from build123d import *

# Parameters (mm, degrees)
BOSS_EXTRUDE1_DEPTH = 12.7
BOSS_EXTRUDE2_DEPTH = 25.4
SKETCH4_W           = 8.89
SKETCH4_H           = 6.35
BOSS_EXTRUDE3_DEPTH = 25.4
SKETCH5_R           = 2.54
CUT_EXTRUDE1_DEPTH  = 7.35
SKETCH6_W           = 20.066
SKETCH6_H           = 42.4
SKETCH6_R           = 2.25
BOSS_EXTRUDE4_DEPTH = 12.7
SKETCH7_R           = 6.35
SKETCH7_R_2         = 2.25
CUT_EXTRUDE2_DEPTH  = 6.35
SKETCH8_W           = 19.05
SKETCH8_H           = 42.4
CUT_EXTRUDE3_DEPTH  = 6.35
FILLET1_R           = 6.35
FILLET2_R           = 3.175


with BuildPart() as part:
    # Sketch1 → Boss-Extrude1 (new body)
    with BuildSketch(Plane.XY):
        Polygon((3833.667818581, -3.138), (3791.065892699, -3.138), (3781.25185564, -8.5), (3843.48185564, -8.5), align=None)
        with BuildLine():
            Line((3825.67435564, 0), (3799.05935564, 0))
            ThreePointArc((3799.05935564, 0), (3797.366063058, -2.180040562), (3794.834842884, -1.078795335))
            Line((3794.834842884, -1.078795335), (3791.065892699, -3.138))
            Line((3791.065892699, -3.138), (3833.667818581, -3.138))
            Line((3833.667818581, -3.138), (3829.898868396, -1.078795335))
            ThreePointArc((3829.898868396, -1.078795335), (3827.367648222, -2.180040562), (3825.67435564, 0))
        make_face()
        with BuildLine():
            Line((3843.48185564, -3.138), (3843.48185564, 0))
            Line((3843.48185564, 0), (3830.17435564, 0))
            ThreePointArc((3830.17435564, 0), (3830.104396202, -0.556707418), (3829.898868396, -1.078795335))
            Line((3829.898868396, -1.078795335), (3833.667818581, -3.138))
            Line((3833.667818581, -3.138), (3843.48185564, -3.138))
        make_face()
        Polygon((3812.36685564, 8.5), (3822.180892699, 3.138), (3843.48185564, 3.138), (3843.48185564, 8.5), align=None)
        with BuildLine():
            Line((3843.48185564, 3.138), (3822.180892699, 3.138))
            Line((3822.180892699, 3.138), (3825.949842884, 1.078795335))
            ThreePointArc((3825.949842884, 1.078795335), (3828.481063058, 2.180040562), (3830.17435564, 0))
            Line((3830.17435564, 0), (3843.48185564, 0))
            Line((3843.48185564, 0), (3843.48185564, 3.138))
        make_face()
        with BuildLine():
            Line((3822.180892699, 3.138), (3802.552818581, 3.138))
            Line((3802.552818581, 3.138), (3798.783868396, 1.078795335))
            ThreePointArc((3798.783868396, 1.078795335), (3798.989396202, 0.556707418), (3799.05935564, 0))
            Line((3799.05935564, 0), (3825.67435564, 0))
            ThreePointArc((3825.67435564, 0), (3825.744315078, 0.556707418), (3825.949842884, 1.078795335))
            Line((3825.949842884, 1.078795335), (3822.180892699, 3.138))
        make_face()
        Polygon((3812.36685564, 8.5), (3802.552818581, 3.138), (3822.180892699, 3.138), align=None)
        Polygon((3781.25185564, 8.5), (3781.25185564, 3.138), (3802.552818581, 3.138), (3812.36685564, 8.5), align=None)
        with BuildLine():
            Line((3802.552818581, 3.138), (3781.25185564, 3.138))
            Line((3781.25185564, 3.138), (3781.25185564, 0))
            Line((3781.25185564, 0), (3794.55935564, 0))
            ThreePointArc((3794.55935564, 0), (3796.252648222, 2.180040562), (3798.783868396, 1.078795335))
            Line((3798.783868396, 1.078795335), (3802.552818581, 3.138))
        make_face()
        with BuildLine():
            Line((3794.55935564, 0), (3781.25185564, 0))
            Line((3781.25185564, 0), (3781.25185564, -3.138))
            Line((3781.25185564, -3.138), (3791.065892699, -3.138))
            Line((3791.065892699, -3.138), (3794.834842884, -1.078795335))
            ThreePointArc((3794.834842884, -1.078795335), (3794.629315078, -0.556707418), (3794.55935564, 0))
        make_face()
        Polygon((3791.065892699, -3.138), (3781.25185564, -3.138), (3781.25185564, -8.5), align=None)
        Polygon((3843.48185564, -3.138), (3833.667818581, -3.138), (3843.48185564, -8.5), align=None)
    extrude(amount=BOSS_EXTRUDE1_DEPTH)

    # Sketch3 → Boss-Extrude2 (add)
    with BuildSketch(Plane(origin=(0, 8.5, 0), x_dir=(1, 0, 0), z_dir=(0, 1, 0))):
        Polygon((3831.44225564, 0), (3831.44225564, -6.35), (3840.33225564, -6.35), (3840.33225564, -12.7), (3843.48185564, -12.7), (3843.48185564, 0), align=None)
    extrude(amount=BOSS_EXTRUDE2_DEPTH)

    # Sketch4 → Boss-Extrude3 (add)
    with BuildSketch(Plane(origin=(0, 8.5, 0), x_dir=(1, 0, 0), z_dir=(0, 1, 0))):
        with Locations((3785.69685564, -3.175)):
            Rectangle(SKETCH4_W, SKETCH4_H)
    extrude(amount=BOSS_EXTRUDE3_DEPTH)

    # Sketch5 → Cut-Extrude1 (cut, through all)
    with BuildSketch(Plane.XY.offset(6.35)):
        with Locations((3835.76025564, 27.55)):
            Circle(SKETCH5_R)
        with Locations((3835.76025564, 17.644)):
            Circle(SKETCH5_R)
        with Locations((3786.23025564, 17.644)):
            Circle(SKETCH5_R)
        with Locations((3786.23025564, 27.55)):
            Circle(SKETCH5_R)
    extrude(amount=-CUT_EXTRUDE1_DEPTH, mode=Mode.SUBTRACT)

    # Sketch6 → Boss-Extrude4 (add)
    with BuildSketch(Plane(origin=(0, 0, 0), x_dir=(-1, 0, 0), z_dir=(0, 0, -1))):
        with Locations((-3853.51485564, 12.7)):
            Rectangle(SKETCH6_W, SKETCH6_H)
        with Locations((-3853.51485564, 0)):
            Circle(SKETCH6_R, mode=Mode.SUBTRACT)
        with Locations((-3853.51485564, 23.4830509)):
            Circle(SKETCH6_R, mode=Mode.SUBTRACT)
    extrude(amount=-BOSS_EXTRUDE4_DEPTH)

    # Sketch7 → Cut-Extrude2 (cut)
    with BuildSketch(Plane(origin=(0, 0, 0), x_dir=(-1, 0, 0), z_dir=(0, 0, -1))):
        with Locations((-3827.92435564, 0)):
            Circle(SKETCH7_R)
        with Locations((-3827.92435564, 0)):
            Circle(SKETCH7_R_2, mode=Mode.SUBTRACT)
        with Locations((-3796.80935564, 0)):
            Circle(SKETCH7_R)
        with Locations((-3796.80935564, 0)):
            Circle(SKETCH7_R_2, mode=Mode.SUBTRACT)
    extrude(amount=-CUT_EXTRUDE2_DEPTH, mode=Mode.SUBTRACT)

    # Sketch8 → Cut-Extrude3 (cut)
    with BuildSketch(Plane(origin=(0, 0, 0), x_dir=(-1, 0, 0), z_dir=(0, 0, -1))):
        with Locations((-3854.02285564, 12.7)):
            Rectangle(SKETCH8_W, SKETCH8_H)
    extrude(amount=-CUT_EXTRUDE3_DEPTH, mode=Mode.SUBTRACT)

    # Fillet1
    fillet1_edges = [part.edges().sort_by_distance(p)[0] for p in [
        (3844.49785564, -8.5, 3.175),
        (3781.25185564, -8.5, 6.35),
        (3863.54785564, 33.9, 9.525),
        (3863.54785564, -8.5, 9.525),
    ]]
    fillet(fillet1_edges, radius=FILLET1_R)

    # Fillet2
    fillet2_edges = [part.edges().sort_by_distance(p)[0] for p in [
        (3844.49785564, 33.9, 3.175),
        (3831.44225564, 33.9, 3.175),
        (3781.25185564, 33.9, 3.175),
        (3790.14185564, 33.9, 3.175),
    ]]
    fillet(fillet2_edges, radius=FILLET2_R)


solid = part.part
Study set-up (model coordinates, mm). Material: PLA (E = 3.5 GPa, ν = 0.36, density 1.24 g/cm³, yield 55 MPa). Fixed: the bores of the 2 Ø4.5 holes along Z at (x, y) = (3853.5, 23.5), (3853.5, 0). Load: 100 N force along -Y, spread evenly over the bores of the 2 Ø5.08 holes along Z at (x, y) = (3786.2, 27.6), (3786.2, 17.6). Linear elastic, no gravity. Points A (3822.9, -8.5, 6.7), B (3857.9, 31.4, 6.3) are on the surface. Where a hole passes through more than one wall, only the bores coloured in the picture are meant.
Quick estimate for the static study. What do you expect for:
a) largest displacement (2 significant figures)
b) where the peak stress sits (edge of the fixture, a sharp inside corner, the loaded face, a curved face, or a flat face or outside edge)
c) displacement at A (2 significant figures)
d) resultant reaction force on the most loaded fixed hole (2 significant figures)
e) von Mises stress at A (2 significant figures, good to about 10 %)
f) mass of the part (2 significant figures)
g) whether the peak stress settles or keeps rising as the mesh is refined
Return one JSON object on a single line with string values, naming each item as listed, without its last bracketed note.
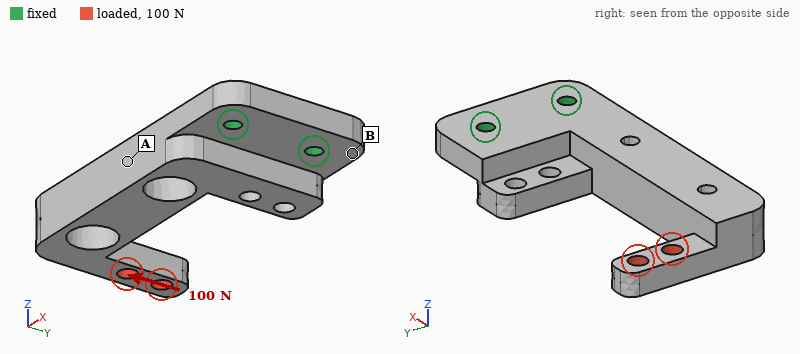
{"largest displacement": "0.80 mm", "where the peak stress sits": "a sharp inside corner", "displacement at A": "0.17 mm", "resultant reaction force on the most loaded fixed hole": "290 N", "von Mises stress at A": "6.1 MPa", "mass of the part": "25 g", "whether the peak stress settles or keeps rising as the mesh is refined": "keeps rising"}
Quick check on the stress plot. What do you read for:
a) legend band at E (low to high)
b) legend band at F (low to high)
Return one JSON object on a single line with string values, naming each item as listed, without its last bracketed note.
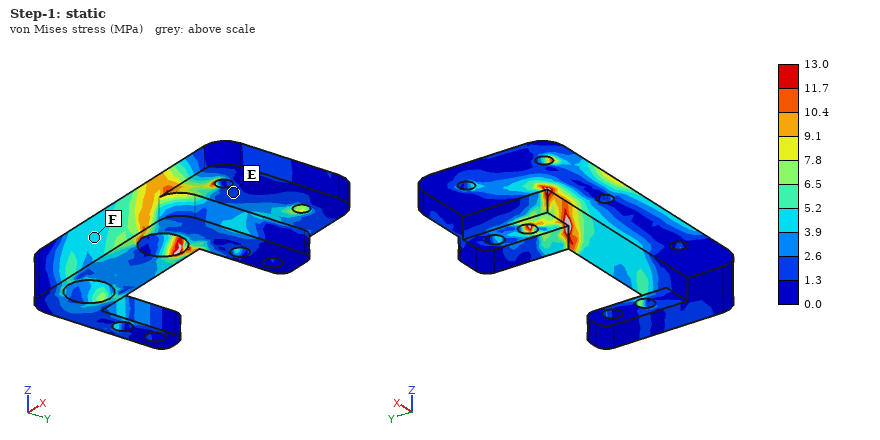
{"legend band at E": "1.3 to 2.6 MPa", "legend band at F": "3.9 to 5.2 MPa"}
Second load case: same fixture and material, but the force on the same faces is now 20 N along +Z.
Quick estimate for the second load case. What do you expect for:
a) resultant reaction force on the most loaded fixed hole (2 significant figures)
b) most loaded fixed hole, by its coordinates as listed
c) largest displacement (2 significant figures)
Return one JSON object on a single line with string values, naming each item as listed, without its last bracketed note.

{"resultant reaction force on the most loaded fixed hole": "19 N", "most loaded fixed hole, by its coordinates as listed": "(3853.5, 23.5)", "largest displacement": "0.90 mm"}
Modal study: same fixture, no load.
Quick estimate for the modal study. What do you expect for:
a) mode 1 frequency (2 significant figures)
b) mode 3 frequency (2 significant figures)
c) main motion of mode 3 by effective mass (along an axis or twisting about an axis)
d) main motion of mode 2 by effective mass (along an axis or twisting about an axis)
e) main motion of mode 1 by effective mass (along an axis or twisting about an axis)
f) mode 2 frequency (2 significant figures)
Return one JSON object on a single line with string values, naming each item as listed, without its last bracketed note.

{"mode 1 frequency": "360 Hz", "mode 3 frequency": "1300 Hz", "main motion of mode 3 by effective mass": "twisting about X", "main motion of mode 2 by effective mass": "along Y", "main motion of mode 1 by effective mass": "along Z", "mode 2 frequency": "830 Hz"}
